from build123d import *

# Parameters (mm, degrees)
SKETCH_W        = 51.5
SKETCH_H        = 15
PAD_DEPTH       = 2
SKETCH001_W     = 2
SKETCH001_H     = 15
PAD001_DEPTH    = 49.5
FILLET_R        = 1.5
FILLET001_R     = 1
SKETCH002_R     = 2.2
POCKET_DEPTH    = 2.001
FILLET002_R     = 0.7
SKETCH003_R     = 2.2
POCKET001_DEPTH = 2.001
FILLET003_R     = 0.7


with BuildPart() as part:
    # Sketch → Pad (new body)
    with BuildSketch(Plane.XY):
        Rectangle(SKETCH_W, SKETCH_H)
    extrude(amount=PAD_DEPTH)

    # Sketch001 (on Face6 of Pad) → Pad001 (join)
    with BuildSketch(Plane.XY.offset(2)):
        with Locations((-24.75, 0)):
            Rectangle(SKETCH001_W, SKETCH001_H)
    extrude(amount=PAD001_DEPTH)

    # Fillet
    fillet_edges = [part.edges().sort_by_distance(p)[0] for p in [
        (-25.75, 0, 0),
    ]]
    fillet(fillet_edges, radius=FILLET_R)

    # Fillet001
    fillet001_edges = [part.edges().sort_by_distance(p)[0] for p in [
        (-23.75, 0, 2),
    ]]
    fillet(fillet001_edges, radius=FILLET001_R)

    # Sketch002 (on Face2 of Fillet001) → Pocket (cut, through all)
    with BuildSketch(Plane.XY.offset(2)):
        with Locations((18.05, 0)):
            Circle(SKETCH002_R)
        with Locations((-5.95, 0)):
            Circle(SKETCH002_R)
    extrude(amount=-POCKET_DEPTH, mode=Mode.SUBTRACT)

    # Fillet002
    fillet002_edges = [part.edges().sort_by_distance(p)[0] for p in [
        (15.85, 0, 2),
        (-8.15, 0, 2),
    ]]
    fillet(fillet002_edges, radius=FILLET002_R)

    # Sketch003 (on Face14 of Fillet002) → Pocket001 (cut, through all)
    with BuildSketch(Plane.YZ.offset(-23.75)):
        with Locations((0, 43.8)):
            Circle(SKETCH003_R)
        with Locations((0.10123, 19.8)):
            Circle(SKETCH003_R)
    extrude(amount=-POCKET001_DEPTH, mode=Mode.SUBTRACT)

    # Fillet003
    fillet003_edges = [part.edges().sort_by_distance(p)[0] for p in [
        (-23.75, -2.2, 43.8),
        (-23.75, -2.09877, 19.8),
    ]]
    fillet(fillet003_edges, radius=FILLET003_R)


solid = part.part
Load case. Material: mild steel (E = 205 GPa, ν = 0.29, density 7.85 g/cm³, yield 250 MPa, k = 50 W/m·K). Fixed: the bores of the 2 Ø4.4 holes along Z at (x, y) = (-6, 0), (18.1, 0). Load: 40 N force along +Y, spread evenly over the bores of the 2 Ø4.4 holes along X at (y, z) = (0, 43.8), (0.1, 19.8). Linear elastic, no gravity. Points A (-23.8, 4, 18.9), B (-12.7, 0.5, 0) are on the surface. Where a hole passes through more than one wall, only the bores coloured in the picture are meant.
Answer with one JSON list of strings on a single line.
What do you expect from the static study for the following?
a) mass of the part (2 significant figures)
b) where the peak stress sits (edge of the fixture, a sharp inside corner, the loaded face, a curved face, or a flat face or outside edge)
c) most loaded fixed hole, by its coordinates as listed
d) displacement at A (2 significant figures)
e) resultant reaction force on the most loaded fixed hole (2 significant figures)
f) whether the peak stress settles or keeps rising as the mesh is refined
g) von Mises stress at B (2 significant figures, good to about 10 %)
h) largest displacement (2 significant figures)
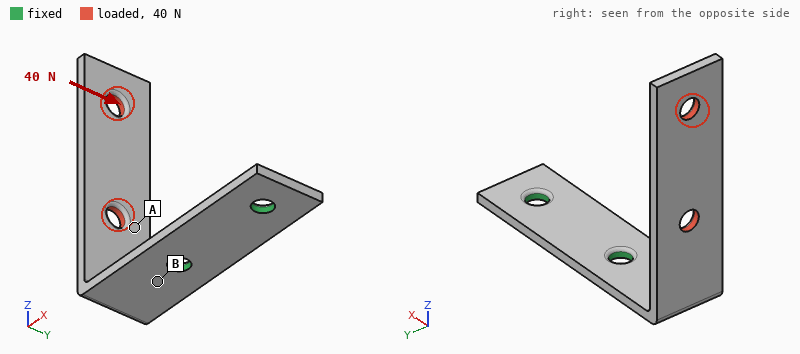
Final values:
["23 g", "edge of the fixture", "(-6, 0)", "0.12 mm", "54 N", "keeps rising", "100 MPa", "0.34 mm"]
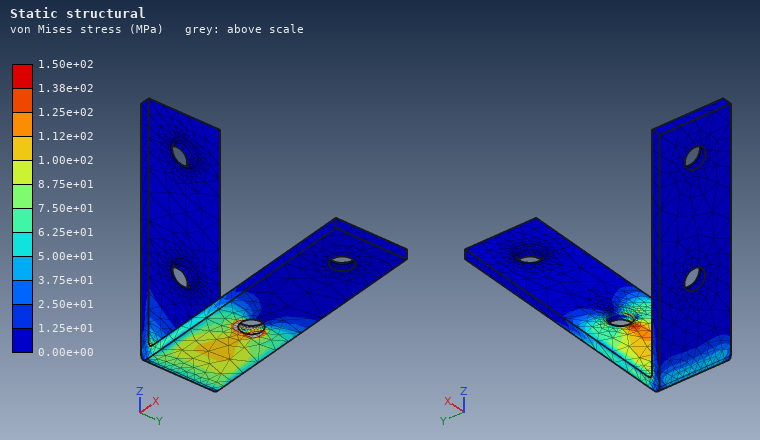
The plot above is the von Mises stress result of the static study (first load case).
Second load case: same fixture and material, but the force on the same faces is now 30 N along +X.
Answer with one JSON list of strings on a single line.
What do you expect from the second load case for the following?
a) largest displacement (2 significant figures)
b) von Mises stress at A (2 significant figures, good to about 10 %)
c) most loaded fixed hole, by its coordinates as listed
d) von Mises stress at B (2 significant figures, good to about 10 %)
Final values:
["0.69 mm", "56 MPa", "(18.1, 0)", "83 MPa"]
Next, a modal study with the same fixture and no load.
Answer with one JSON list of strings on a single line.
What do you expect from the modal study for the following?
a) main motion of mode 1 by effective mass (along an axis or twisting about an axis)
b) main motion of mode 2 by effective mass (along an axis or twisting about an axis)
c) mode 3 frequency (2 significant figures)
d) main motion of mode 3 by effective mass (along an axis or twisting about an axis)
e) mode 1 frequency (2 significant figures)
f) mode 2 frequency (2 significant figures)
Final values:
["along X", "along Y", "1800 Hz", "along Z", "420 Hz", "690 Hz"]
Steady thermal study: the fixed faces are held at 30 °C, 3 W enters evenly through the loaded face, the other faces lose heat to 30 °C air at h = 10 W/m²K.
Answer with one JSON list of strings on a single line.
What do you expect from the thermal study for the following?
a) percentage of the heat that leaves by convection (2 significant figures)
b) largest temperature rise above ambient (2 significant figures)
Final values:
["33 %", "73 K"]
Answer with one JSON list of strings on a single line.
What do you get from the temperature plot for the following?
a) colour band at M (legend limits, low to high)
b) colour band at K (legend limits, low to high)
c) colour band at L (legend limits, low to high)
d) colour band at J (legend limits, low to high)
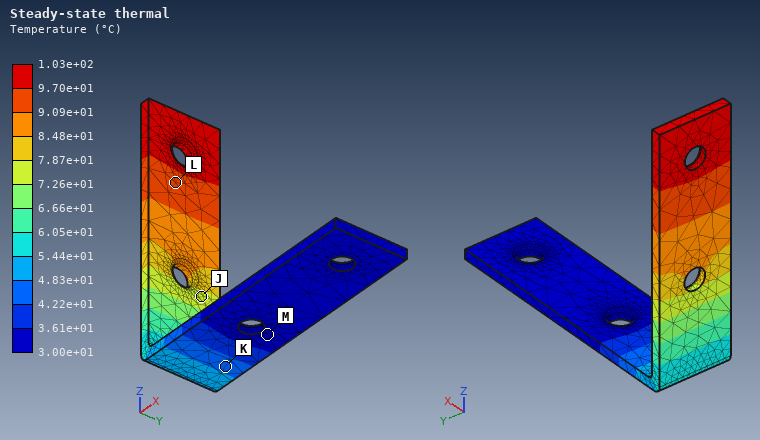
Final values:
["3.00e+01 to 3.61e+01 °C", "4.22e+01 to 4.83e+01 °C", "9.09e+01 to 9.70e+01 °C", "7.26e+01 to 7.87e+01 °C"]
